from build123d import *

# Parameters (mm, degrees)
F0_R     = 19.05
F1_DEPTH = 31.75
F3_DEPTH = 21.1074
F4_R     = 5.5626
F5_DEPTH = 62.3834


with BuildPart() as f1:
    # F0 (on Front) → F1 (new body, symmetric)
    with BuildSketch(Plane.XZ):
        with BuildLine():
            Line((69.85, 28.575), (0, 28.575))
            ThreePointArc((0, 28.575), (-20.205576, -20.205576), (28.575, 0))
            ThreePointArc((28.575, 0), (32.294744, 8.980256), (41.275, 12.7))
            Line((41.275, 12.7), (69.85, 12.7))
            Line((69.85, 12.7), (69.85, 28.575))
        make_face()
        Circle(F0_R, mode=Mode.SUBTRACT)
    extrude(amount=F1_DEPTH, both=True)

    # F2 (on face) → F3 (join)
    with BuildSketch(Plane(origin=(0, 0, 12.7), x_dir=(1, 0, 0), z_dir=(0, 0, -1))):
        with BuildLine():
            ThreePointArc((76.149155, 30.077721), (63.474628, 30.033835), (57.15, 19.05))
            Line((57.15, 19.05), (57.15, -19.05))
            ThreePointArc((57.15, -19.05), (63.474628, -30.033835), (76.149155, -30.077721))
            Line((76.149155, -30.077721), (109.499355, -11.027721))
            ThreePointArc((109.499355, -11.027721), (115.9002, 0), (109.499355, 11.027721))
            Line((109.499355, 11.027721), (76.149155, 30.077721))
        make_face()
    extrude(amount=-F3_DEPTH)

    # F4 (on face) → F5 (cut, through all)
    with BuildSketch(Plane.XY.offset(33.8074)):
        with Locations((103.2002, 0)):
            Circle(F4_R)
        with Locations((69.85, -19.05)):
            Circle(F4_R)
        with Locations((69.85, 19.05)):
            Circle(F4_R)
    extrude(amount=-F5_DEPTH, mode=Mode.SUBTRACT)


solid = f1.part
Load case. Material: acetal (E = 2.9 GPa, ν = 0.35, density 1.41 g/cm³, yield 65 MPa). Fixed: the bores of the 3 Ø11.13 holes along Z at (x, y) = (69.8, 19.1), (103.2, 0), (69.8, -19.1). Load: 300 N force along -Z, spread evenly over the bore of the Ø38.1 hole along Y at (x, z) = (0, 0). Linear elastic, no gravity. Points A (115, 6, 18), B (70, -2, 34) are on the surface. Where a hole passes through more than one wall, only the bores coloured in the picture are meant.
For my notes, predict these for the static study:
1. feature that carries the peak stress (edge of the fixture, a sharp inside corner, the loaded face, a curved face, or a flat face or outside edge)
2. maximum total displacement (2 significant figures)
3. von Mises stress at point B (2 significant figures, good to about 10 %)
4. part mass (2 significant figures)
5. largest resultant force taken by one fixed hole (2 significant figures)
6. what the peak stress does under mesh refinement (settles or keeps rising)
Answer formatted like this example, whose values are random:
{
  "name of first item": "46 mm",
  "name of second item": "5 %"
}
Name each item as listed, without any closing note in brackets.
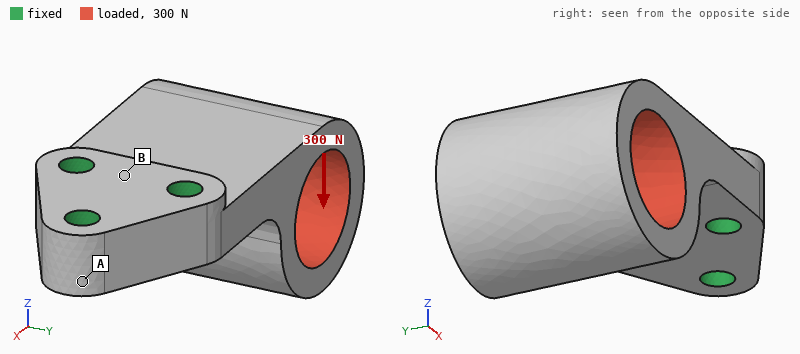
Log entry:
{
  "feature that carries the peak stress": "edge of the fixture",
  "maximum total displacement": "0.72 mm",
  "von Mises stress at point B": "1.7 MPa",
  "part mass": "260 g",
  "largest resultant force taken by one fixed hole": "190 N",
  "what the peak stress does under mesh refinement": "keeps rising"
}
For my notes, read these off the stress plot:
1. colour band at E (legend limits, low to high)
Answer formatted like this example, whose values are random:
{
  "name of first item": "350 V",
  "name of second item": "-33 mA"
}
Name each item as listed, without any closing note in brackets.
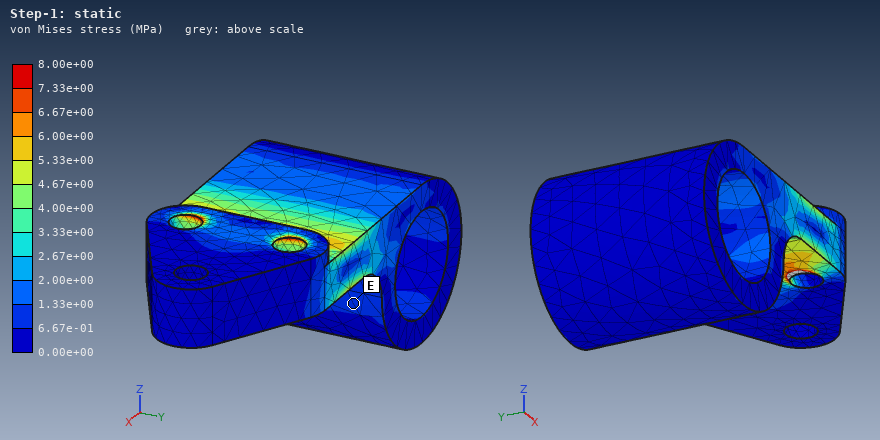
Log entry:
{
  "colour band at E": "6.67e-01 to 1.33e+00 MPa"
}
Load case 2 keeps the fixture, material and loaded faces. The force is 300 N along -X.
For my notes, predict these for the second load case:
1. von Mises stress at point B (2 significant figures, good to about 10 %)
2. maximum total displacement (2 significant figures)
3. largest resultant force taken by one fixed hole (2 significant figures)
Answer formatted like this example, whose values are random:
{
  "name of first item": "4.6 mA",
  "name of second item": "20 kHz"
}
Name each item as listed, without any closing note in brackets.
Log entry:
{
  "von Mises stress at point B": "0.52 MPa",
  "maximum total displacement": "0.33 mm",
  "largest resultant force taken by one fixed hole": "140 N"
}
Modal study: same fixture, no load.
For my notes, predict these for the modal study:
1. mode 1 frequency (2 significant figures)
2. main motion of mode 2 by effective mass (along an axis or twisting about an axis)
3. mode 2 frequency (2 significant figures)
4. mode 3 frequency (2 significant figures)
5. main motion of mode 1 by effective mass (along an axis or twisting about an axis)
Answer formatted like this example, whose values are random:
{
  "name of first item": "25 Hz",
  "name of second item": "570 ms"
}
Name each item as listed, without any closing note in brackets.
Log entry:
{
  "mode 1 frequency": "300 Hz",
  "main motion of mode 2 by effective mass": "along Y",
  "mode 2 frequency": "740 Hz",
  "mode 3 frequency": "1200 Hz",
  "main motion of mode 1 by effective mass": "along Z"
}
